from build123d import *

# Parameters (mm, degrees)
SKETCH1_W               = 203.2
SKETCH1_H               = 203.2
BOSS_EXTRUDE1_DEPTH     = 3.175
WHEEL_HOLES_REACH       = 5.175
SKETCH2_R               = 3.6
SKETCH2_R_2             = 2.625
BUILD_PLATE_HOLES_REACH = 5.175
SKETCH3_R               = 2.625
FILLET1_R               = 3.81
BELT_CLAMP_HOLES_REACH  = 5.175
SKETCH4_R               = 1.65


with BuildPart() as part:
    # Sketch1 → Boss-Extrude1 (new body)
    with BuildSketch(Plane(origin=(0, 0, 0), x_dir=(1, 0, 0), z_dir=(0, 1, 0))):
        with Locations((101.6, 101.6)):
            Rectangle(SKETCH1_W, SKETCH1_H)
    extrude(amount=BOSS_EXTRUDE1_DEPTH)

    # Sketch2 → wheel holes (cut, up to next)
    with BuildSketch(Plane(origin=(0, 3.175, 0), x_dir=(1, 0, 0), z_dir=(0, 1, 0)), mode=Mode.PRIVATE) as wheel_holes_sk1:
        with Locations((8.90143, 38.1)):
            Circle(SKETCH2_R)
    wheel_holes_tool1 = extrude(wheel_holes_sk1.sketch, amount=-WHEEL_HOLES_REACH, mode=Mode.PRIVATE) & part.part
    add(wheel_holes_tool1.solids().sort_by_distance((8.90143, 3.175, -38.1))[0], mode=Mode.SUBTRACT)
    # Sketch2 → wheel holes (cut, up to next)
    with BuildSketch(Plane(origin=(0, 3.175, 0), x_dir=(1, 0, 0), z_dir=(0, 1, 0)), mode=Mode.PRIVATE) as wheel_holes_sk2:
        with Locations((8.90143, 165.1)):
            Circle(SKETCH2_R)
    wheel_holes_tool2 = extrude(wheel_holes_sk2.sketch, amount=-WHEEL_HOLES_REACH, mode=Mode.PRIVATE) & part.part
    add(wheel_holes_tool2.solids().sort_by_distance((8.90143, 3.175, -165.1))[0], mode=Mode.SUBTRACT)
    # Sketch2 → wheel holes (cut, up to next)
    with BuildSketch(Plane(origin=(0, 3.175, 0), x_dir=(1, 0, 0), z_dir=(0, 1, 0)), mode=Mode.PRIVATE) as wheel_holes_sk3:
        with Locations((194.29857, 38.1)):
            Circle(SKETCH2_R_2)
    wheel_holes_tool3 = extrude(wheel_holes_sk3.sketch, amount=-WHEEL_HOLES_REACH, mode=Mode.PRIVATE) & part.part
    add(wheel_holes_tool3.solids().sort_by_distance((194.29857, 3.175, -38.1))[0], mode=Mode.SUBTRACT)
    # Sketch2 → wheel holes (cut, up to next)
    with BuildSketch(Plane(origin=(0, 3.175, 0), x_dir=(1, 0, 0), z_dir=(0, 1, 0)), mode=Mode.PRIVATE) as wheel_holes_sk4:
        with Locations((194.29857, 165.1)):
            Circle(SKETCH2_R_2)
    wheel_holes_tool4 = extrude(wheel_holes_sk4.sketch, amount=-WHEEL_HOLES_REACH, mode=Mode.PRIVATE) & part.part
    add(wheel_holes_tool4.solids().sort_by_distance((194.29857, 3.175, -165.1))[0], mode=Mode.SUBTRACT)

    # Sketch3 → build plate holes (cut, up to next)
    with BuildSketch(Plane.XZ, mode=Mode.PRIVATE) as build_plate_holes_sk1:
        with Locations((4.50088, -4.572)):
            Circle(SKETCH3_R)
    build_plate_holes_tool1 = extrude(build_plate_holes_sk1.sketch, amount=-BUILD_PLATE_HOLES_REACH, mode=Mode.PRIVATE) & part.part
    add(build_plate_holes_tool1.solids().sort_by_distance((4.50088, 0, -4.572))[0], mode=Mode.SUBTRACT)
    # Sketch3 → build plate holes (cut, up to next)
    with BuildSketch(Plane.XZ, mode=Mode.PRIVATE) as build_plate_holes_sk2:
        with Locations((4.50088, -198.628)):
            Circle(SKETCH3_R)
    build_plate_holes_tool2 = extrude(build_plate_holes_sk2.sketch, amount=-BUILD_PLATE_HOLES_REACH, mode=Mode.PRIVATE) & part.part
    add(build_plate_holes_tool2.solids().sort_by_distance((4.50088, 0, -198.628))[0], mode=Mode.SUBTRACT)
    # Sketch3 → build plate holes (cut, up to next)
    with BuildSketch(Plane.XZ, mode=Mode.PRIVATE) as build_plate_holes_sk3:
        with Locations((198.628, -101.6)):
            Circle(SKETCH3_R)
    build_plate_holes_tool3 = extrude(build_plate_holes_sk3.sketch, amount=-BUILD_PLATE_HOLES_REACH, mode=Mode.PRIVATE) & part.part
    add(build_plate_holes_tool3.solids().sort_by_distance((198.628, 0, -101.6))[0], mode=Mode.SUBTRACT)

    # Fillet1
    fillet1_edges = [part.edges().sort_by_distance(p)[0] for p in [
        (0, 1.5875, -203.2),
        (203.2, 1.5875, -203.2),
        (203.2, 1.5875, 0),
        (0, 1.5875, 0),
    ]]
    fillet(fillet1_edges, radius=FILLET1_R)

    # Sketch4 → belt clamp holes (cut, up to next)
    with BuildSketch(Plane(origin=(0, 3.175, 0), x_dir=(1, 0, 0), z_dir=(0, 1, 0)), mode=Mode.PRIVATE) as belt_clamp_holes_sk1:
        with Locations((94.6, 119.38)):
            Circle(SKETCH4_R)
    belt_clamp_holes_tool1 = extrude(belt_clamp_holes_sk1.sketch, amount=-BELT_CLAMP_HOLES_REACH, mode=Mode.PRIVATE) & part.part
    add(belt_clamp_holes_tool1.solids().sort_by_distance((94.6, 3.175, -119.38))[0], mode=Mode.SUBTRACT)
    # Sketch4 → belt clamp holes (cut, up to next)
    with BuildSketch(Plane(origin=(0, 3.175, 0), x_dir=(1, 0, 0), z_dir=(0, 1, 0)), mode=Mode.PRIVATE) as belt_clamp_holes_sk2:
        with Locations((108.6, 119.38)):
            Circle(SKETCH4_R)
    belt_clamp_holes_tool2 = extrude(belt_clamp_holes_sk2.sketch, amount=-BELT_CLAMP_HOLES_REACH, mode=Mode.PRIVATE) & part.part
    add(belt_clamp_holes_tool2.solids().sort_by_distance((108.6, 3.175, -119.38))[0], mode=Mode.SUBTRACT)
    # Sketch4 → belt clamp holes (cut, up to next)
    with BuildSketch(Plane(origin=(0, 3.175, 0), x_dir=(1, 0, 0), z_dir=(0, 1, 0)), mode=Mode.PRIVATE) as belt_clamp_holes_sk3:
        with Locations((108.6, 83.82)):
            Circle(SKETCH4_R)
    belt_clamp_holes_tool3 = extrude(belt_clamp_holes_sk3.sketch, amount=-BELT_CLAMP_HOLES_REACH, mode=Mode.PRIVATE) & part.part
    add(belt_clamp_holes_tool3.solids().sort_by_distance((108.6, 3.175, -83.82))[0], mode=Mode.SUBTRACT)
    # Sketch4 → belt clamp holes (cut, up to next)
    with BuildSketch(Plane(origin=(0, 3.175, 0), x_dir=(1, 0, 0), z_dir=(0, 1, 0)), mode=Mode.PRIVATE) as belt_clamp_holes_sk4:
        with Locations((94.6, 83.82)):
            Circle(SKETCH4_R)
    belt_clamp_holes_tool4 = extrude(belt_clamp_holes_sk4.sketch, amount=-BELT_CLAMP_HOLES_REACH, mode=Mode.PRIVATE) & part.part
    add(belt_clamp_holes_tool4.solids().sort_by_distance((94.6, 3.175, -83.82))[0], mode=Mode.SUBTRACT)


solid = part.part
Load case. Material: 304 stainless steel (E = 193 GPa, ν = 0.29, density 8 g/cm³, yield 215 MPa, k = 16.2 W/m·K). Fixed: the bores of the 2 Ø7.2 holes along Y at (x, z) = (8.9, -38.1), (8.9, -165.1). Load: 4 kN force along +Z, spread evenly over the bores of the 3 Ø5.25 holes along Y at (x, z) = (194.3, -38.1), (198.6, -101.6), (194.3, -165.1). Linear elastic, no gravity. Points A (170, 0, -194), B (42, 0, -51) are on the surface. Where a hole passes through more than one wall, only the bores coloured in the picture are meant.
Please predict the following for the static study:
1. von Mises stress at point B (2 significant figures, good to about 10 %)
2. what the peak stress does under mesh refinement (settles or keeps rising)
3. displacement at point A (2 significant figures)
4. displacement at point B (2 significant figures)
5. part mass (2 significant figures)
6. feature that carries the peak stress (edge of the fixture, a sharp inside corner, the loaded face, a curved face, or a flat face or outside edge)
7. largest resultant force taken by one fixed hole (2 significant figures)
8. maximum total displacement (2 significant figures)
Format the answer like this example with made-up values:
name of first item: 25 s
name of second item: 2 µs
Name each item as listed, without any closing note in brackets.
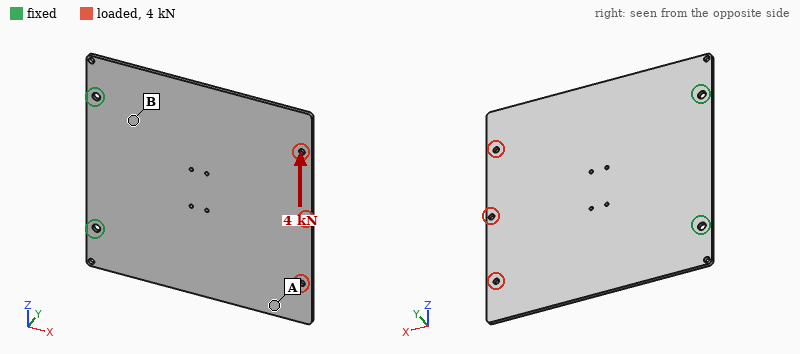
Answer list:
von Mises stress at point B: 33 MPa
what the peak stress does under mesh refinement: keeps rising
displacement at point A: 62 µm
displacement at point B: 13 µm
part mass: 1.0 kg
feature that carries the peak stress: edge of the fixture
largest resultant force taken by one fixed hole: 6.1 kN
maximum total displacement: 74 µm
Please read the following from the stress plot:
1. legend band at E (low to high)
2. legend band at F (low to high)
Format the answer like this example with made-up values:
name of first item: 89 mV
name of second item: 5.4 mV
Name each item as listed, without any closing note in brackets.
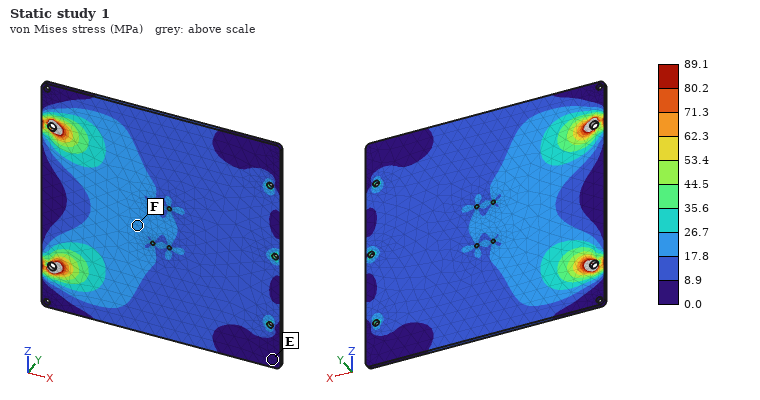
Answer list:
legend band at E: 0.0 to 8.9 MPa
legend band at F: 17.8 to 26.7 MPa
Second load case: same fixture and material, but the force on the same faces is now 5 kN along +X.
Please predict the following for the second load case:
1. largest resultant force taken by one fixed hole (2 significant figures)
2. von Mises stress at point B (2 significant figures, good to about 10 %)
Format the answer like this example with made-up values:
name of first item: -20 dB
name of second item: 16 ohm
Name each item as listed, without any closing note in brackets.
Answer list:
largest resultant force taken by one fixed hole: 2.5 kN
von Mises stress at point B: 14 MPa
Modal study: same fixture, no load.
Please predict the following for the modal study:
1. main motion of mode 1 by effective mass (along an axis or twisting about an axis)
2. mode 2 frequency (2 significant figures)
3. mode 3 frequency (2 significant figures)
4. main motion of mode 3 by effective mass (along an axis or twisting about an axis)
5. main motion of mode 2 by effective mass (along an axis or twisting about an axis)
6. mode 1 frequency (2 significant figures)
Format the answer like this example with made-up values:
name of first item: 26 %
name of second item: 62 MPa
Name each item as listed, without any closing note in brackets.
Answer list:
main motion of mode 1 by effective mass: along Y
mode 2 frequency: 160 Hz
mode 3 frequency: 380 Hz
main motion of mode 3 by effective mass: along Y
main motion of mode 2 by effective mass: twisting about X
mode 1 frequency: 59 Hz
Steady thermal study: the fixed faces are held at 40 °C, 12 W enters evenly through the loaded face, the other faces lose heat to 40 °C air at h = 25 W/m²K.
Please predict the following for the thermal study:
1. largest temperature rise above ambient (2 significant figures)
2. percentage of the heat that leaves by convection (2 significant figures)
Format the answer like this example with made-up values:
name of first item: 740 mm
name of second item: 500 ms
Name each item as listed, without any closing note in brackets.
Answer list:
largest temperature rise above ambient: 65 K
percentage of the heat that leaves by convection: 100 %
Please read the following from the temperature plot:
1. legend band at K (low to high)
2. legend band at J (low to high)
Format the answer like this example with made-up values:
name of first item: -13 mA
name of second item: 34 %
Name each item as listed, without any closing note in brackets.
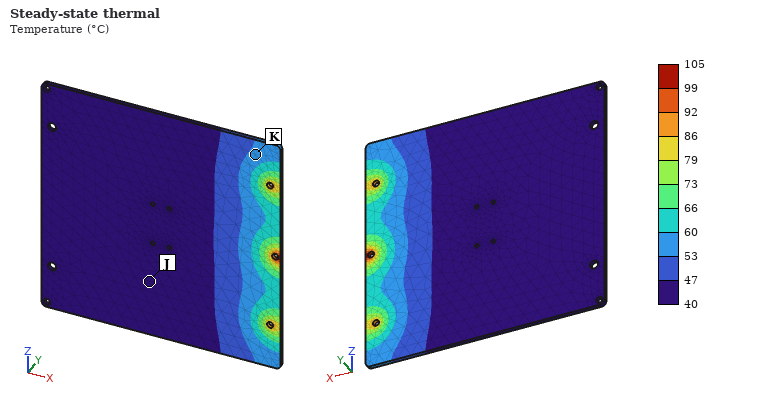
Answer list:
legend band at K: 53 to 60 °C
legend band at J: 40 to 47 °C
